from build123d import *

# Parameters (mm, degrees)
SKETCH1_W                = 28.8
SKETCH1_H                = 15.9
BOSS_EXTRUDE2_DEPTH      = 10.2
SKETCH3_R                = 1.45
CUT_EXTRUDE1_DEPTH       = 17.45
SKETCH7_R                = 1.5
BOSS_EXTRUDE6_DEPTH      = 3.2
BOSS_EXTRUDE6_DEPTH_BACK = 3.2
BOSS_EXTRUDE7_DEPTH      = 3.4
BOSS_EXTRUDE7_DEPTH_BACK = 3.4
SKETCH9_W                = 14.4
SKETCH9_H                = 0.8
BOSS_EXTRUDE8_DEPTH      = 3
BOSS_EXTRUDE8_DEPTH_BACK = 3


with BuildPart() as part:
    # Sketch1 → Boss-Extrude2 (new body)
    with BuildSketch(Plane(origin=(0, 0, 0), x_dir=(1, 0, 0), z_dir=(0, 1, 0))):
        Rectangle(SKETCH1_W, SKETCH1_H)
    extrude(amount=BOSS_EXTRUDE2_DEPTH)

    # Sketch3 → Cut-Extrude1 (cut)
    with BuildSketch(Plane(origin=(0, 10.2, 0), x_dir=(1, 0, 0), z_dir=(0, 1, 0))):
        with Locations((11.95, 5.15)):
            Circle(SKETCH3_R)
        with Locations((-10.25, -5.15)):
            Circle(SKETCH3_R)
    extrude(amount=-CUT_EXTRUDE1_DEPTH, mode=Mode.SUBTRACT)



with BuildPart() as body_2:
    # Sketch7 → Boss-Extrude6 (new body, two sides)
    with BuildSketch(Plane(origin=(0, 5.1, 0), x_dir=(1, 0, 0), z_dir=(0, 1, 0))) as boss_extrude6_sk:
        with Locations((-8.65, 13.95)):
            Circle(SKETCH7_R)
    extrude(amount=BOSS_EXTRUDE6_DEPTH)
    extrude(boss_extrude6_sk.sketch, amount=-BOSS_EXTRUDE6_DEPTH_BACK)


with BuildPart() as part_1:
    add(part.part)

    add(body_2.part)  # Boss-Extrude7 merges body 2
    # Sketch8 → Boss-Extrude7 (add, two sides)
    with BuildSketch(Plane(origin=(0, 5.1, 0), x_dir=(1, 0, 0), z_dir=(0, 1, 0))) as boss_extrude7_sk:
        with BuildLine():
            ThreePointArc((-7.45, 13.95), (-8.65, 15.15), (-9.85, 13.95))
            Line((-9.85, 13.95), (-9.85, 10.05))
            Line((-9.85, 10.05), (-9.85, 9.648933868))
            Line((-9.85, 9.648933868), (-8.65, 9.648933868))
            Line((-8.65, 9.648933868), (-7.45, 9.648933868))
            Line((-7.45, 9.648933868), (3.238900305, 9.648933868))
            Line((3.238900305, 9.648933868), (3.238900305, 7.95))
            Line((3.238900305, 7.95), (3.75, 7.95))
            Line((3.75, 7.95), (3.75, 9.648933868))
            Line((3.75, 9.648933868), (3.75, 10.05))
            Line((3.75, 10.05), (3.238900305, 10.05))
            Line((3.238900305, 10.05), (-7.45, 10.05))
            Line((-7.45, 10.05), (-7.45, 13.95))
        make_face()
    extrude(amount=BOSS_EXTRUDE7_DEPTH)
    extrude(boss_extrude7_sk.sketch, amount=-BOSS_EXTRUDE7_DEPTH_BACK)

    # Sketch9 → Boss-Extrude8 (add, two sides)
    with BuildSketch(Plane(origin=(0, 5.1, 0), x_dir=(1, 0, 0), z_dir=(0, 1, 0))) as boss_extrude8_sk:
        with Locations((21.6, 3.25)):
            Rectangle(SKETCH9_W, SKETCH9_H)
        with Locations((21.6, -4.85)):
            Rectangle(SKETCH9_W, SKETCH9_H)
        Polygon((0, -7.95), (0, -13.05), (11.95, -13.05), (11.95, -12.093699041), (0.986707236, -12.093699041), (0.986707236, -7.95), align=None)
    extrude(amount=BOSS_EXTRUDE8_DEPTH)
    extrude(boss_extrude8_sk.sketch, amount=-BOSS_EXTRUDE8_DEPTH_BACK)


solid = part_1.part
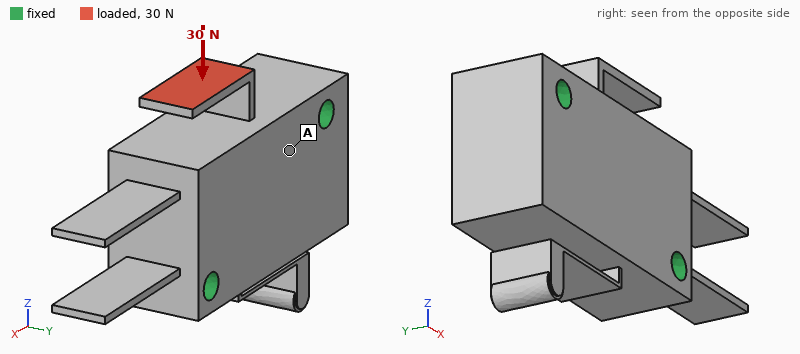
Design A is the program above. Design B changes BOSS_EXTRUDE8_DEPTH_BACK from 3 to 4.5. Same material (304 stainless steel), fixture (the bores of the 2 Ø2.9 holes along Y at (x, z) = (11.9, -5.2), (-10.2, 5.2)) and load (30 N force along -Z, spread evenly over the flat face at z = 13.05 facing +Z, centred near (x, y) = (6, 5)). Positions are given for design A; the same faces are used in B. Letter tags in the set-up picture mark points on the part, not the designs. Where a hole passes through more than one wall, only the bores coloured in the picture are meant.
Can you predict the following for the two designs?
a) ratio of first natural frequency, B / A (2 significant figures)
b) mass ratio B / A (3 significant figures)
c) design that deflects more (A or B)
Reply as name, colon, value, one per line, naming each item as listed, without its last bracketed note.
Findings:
ratio of first natural frequency, B / A: 1.0
mass ratio B / A: 1.01
design that deflects more: A
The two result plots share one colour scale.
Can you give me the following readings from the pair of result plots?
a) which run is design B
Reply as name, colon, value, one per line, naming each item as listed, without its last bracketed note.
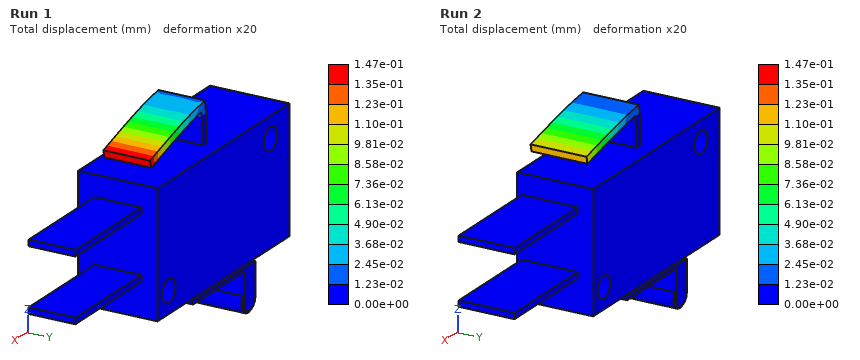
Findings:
which run is design B: Run 2
